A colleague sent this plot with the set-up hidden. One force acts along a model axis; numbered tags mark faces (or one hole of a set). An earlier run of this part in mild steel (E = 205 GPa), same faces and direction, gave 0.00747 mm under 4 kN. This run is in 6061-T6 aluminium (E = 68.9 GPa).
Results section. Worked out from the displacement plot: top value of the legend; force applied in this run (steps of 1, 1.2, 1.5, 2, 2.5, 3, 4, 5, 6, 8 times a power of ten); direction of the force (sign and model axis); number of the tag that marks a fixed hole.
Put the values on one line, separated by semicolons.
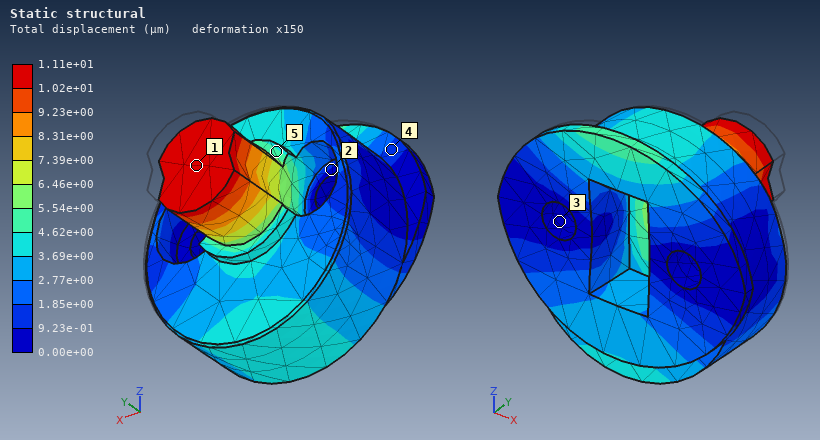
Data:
1.11e+01 µm; 2 kN; -Y; 3
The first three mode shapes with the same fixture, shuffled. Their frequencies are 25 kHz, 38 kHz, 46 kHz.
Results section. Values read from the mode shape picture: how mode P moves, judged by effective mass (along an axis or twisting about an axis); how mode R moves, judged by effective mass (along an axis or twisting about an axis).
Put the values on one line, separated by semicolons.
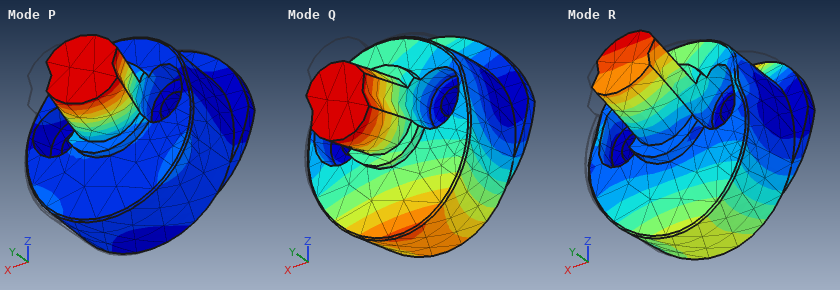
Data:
along X; along Y
